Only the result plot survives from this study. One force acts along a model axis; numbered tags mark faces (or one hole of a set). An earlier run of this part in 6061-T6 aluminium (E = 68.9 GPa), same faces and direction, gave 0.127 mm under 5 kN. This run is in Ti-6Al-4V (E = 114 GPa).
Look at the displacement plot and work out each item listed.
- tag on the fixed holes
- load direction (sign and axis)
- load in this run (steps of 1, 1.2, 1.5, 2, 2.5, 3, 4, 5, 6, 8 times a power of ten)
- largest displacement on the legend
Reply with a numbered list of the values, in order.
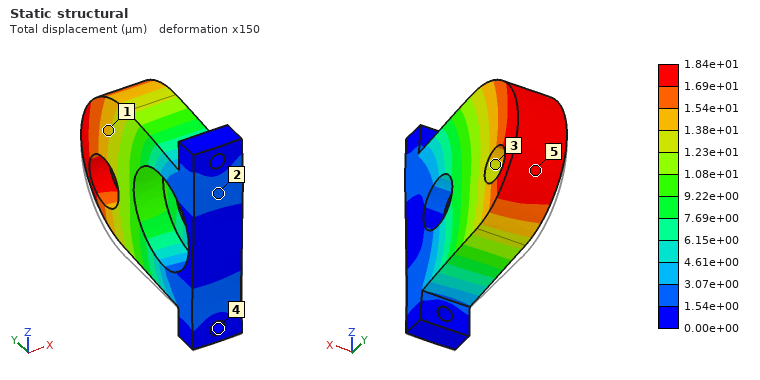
1. 4
2. +Z
3. 1.2 kN
4. 1.84e+01 µm
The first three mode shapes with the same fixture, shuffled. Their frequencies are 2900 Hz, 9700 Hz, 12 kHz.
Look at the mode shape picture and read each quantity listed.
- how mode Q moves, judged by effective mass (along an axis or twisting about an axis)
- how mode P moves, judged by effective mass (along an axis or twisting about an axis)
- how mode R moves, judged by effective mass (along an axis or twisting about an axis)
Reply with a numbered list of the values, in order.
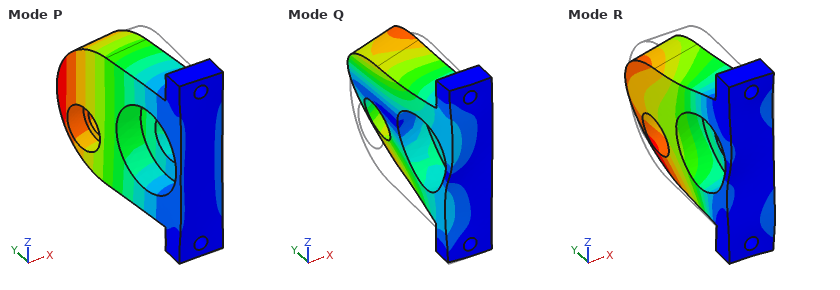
1. along Z
2. along X
3. along Z
